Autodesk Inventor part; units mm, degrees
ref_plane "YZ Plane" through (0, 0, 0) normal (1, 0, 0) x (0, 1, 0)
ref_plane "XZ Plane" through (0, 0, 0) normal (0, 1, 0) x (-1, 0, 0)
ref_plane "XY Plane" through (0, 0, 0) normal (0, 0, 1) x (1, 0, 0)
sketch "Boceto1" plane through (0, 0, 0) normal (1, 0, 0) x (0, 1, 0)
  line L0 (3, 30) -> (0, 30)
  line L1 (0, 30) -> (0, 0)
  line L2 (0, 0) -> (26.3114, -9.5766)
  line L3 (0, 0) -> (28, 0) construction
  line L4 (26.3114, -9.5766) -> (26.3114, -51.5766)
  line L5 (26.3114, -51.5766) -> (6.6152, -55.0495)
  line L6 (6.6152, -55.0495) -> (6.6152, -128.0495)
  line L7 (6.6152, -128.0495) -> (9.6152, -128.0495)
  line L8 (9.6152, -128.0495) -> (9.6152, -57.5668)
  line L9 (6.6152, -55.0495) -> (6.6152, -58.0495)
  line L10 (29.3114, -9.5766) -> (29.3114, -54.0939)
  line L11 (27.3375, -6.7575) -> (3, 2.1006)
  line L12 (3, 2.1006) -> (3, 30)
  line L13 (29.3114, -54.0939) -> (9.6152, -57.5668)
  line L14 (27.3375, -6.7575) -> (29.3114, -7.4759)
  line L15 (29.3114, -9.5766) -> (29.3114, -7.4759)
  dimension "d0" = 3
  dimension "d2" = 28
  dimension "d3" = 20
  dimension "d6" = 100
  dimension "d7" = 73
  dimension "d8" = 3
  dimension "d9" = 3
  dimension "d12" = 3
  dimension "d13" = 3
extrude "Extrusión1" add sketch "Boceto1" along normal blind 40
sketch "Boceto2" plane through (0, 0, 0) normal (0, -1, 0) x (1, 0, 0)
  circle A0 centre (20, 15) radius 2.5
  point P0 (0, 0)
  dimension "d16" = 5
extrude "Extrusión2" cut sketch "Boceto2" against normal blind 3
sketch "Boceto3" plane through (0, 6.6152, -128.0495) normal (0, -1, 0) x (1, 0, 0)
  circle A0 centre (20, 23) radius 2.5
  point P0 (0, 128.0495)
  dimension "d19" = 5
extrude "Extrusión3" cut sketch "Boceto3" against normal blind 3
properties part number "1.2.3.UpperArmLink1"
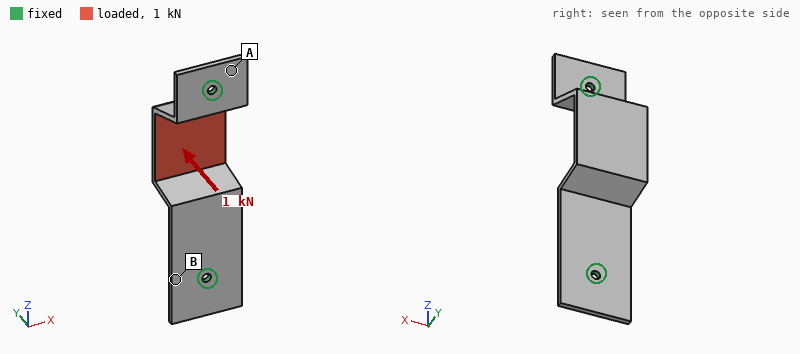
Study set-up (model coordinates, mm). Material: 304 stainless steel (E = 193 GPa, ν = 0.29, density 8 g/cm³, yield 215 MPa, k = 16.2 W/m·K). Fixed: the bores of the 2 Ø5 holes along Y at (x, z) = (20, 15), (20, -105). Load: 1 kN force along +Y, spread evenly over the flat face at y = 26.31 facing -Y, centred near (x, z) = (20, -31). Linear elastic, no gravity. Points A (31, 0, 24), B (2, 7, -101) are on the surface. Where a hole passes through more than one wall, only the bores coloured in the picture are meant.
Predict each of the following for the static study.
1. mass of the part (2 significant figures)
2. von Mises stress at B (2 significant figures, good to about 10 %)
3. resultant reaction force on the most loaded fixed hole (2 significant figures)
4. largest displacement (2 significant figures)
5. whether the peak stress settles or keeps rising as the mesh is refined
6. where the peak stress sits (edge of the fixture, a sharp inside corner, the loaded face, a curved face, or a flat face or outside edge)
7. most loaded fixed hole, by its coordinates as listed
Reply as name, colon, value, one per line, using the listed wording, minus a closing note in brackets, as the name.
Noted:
mass of the part: 180 g
von Mises stress at B: 75 MPa
resultant reaction force on the most loaded fixed hole: 850 N
largest displacement: 0.25 mm
whether the peak stress settles or keeps rising as the mesh is refined: keeps rising
where the peak stress sits: edge of the fixture
most loaded fixed hole, by its coordinates as listed: (20, 15)
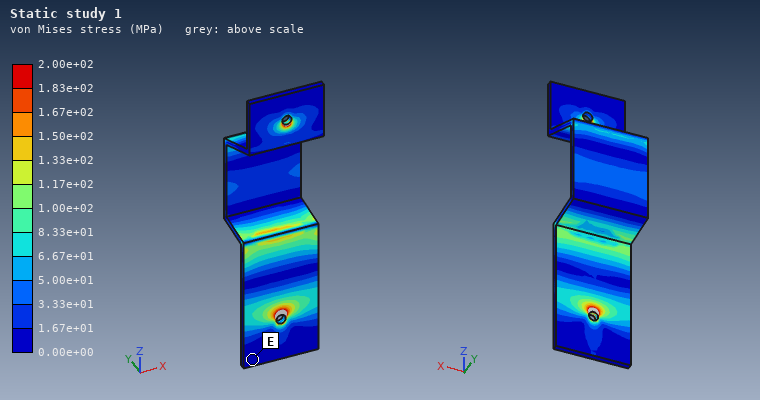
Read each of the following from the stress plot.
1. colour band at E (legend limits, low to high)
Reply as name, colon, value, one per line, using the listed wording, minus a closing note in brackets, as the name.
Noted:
colour band at E: 0.00e+00 to 1.67e+01 MPa
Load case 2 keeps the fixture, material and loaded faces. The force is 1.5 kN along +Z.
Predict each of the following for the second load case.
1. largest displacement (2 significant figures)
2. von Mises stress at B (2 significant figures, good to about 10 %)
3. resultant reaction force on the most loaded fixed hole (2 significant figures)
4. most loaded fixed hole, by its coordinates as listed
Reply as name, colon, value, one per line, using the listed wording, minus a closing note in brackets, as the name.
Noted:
largest displacement: 0.13 mm
von Mises stress at B: 42 MPa
resultant reaction force on the most loaded fixed hole: 970 N
most loaded fixed hole, by its coordinates as listed: (20, -105)
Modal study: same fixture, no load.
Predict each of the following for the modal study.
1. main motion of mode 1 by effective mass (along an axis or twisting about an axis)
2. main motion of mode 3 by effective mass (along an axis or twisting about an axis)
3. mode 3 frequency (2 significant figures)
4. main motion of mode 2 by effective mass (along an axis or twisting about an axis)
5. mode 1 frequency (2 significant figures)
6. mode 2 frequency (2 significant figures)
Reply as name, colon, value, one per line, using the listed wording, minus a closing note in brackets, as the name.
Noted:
main motion of mode 1 by effective mass: along Y
main motion of mode 3 by effective mass: along Z
mode 3 frequency: 2400 Hz
main motion of mode 2 by effective mass: along X
mode 1 frequency: 1000 Hz
mode 2 frequency: 1100 Hz
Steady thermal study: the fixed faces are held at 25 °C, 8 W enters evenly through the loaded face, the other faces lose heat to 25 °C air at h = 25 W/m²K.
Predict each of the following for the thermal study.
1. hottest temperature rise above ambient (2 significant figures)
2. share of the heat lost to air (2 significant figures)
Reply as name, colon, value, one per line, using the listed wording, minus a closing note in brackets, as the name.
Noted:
hottest temperature rise above ambient: 55 K
share of the heat lost to air: 82 %
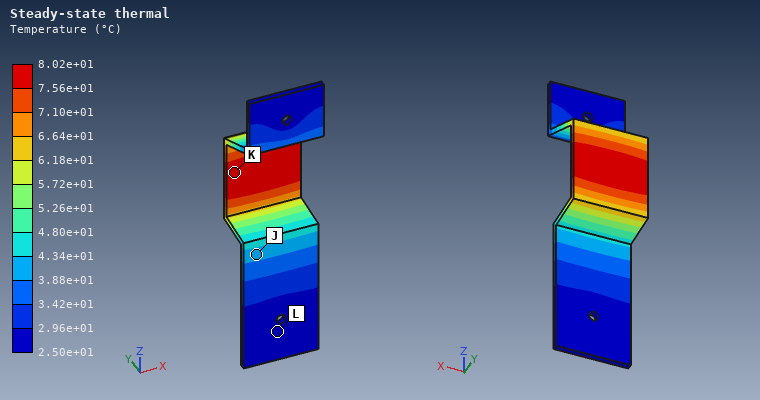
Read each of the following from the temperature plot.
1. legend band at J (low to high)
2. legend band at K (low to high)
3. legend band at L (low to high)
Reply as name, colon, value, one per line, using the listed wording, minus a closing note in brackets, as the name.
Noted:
legend band at J: 3.88e+01 to 4.34e+01 °C
legend band at K: 7.56e+01 to 8.02e+01 °C
legend band at L: 2.50e+01 to 2.96e+01 °C
